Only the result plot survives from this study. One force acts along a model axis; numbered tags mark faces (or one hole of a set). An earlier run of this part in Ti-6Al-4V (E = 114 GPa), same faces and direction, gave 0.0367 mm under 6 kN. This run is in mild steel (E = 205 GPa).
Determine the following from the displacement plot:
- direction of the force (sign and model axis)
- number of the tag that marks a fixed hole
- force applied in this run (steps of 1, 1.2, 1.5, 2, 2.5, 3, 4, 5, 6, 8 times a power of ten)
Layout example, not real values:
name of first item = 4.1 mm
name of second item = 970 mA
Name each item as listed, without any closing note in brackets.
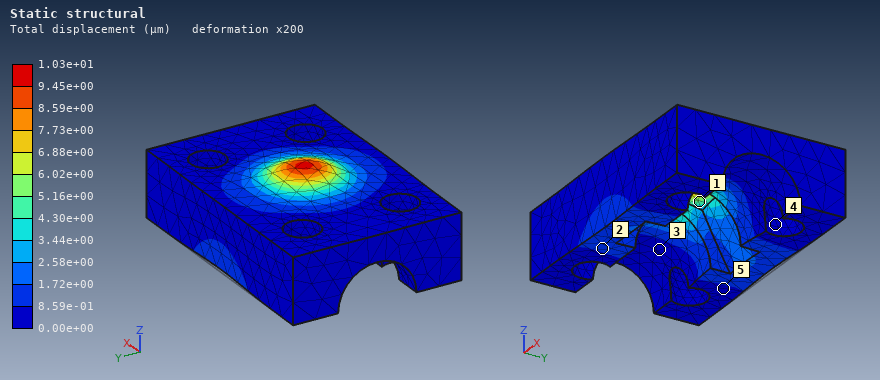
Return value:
direction of the force = +Z
number of the tag that marks a fixed hole = 4
force applied in this run = 3 kN
